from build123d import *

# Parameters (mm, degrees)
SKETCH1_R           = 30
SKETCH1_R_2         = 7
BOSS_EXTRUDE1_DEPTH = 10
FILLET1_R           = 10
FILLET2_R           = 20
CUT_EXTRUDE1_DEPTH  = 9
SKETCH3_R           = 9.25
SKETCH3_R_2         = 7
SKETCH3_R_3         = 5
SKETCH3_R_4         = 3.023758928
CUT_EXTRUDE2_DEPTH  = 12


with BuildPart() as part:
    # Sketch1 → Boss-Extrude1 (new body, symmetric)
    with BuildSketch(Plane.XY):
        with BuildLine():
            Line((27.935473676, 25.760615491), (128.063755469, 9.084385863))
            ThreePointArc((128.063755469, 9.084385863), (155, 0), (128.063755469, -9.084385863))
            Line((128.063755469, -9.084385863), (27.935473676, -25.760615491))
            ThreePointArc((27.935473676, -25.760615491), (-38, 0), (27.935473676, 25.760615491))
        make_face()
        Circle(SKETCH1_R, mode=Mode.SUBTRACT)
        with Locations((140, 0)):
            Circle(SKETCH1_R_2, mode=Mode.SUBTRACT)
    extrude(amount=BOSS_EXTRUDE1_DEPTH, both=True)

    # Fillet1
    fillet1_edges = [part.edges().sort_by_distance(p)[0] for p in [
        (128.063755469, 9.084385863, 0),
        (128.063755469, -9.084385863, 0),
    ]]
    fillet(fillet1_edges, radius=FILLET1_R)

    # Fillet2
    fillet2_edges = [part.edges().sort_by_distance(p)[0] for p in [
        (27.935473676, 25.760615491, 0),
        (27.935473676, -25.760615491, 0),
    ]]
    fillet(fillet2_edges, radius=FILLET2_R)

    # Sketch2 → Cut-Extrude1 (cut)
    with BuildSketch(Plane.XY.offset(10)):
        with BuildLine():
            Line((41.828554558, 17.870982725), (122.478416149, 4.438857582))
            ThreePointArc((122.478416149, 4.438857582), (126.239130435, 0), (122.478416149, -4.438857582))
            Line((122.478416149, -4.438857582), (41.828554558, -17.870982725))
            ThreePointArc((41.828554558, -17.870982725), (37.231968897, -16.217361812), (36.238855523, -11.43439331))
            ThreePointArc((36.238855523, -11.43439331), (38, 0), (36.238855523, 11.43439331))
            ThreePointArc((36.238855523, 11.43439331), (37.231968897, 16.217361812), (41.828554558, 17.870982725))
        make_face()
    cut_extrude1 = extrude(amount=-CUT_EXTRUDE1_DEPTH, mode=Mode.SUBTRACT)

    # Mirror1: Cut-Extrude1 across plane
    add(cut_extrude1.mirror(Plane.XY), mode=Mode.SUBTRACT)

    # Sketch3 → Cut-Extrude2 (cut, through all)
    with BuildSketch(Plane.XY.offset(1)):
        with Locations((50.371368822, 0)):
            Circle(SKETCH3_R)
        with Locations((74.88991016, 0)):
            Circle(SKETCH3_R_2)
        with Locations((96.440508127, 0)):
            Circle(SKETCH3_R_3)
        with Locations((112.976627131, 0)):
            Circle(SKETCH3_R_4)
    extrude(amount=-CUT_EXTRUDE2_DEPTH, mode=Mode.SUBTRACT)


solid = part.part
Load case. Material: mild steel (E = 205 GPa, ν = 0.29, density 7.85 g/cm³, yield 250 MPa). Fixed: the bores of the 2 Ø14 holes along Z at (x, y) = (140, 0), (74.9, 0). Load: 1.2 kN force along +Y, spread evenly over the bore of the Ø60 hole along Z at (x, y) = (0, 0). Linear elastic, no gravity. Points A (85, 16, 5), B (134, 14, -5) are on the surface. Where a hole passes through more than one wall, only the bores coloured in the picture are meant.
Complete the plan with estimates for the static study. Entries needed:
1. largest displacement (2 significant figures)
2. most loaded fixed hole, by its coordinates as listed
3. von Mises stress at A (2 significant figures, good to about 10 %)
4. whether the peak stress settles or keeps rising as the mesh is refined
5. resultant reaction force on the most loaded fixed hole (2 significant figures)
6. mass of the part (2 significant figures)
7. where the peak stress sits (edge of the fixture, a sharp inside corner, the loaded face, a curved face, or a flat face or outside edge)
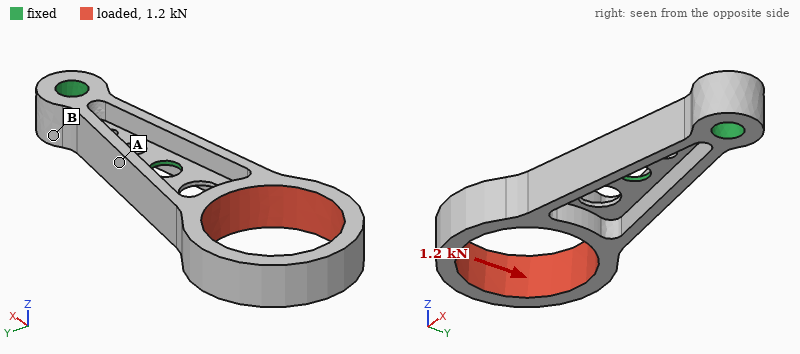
0.12 mm
(74.9, 0)
25 MPa
keeps rising
2.1 kN
550 g
edge of the fixture
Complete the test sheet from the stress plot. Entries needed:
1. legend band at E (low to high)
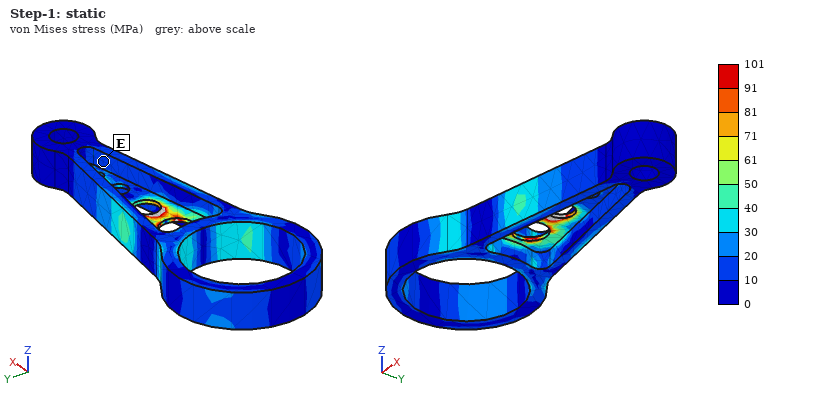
10 to 20 MPa
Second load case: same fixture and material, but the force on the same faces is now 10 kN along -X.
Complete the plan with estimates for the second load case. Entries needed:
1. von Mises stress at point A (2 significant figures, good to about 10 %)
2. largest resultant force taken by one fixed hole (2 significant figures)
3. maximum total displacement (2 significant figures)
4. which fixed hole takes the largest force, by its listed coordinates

28 MPa
6.1 kN
67 µm
(74.9, 0)
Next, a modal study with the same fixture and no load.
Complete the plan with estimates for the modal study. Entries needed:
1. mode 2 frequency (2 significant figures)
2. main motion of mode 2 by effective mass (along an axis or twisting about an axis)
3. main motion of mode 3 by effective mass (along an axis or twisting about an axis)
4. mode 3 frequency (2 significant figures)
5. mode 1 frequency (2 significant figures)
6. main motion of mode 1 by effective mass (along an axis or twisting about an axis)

950 Hz
twisting about X
along Y
1100 Hz
610 Hz
along Z
